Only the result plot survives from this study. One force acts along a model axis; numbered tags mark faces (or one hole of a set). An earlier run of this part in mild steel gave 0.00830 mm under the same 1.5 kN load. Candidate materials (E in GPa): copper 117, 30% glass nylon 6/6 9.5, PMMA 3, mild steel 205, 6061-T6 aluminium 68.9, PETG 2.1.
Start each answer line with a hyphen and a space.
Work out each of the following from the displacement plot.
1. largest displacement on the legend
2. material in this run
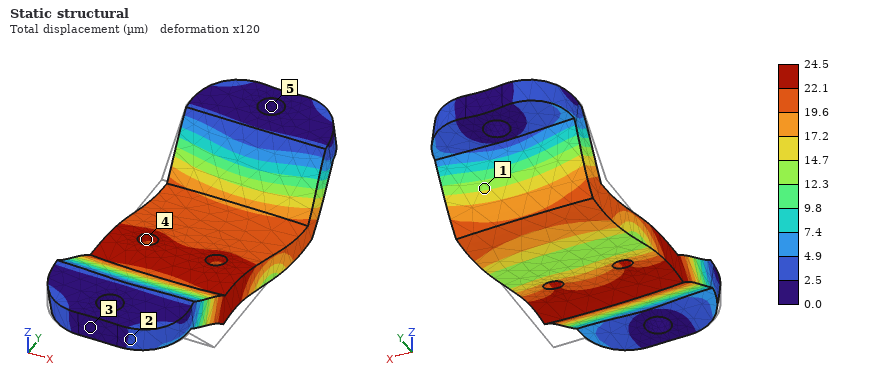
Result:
- 24.5 µm
- 6061-T6 aluminium
